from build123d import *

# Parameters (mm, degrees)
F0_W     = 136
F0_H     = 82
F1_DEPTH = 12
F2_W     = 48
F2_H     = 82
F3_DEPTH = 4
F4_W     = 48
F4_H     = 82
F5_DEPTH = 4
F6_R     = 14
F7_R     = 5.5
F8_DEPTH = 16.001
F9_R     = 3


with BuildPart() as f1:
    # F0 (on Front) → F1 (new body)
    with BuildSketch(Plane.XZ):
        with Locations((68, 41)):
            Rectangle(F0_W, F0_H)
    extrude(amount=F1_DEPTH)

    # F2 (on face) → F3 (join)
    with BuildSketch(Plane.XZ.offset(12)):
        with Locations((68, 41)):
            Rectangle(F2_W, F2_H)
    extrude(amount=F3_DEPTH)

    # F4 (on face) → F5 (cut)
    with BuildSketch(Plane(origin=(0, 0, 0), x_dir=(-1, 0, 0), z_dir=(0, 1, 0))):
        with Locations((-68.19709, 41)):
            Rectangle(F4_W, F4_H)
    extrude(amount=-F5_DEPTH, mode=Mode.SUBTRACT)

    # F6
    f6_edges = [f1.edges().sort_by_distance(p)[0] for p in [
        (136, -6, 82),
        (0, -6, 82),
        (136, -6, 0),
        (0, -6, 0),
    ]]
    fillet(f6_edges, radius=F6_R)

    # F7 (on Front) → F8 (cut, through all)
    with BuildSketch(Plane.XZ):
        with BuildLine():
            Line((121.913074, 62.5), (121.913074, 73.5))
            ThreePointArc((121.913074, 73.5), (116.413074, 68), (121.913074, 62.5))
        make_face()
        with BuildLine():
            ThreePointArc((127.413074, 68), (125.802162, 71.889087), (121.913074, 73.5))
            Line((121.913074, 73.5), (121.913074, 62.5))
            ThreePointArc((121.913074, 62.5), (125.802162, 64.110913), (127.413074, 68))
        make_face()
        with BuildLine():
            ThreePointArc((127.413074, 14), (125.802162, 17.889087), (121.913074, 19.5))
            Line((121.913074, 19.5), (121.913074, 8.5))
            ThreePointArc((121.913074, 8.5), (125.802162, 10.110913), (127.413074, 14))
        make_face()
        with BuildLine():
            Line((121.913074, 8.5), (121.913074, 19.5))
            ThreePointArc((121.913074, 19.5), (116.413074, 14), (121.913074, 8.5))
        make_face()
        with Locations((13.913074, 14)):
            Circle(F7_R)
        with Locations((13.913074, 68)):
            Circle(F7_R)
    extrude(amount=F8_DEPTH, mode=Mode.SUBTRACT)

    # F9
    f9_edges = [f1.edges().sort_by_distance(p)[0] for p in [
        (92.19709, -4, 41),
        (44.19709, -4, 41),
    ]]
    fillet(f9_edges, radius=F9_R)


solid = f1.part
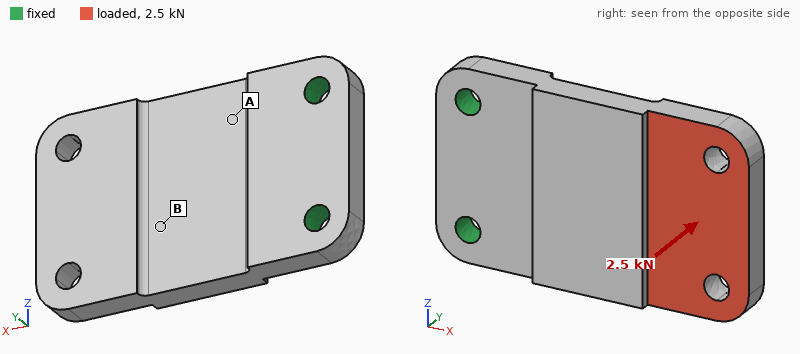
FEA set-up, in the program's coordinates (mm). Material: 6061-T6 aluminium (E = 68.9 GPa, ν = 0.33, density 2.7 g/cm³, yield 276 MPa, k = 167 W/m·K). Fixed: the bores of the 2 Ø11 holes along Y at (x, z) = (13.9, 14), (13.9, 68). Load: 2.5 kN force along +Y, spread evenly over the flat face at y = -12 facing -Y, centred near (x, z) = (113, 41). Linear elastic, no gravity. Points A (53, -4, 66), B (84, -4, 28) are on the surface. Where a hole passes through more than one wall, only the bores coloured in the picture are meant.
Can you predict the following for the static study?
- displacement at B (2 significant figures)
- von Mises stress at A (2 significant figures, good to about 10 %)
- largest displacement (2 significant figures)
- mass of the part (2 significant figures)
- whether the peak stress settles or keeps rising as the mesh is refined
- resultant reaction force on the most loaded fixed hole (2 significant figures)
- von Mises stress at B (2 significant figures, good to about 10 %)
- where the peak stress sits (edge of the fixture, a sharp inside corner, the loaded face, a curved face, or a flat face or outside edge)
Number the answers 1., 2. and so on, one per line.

1. 0.64 mm
2. 76 MPa
3. 1.5 mm
4. 340 g
5. keeps rising
6. 1.3 kN
7. 39 MPa
8. edge of the fixture
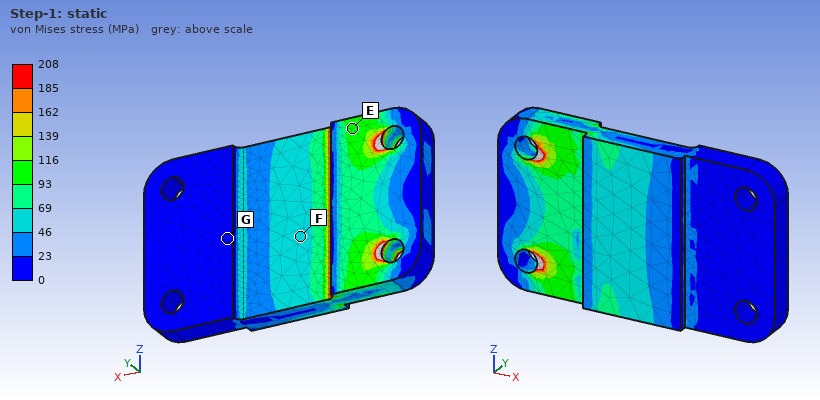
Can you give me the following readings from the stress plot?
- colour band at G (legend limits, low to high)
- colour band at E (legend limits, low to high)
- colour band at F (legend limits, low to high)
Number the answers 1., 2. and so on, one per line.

1. 0 to 23 MPa
2. 93 to 116 MPa
3. 46 to 69 MPa
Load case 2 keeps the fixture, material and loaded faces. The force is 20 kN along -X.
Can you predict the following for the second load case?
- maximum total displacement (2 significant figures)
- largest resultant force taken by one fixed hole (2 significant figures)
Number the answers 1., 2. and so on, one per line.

1. 0.85 mm
2. 10 kN
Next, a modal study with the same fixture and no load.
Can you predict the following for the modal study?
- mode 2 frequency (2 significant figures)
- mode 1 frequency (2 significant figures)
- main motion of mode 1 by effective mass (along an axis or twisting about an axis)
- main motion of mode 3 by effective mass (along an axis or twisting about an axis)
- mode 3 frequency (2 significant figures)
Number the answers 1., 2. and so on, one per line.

1. 2100 Hz
2. 650 Hz
3. along Y
4. along Z
5. 3400 Hz
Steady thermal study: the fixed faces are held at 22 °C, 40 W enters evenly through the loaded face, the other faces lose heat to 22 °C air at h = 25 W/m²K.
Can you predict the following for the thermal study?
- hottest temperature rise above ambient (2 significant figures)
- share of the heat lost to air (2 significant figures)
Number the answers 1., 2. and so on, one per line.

1. 23 K
2. 17 %
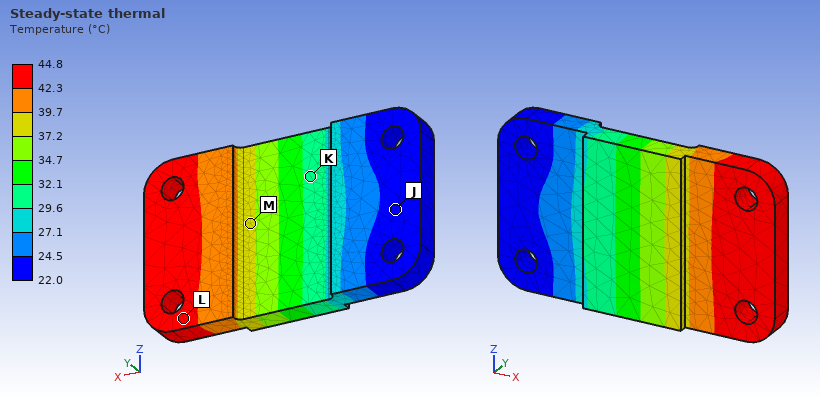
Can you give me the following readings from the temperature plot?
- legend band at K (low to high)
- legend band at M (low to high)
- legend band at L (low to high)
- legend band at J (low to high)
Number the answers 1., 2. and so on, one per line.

1. 29.6 to 32.1 °C
2. 37.2 to 39.7 °C
3. 42.3 to 44.8 °C
4. 22.0 to 24.5 °C
